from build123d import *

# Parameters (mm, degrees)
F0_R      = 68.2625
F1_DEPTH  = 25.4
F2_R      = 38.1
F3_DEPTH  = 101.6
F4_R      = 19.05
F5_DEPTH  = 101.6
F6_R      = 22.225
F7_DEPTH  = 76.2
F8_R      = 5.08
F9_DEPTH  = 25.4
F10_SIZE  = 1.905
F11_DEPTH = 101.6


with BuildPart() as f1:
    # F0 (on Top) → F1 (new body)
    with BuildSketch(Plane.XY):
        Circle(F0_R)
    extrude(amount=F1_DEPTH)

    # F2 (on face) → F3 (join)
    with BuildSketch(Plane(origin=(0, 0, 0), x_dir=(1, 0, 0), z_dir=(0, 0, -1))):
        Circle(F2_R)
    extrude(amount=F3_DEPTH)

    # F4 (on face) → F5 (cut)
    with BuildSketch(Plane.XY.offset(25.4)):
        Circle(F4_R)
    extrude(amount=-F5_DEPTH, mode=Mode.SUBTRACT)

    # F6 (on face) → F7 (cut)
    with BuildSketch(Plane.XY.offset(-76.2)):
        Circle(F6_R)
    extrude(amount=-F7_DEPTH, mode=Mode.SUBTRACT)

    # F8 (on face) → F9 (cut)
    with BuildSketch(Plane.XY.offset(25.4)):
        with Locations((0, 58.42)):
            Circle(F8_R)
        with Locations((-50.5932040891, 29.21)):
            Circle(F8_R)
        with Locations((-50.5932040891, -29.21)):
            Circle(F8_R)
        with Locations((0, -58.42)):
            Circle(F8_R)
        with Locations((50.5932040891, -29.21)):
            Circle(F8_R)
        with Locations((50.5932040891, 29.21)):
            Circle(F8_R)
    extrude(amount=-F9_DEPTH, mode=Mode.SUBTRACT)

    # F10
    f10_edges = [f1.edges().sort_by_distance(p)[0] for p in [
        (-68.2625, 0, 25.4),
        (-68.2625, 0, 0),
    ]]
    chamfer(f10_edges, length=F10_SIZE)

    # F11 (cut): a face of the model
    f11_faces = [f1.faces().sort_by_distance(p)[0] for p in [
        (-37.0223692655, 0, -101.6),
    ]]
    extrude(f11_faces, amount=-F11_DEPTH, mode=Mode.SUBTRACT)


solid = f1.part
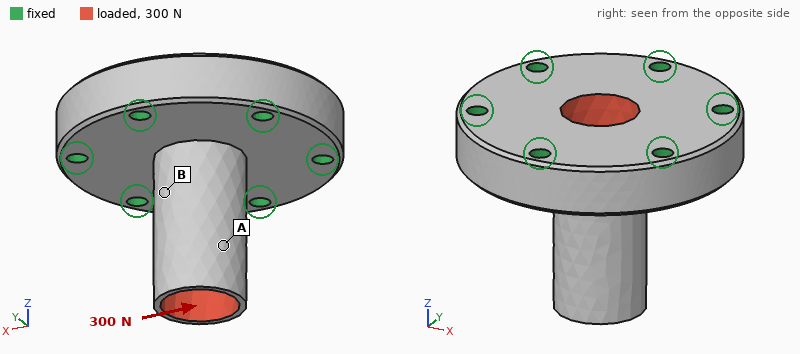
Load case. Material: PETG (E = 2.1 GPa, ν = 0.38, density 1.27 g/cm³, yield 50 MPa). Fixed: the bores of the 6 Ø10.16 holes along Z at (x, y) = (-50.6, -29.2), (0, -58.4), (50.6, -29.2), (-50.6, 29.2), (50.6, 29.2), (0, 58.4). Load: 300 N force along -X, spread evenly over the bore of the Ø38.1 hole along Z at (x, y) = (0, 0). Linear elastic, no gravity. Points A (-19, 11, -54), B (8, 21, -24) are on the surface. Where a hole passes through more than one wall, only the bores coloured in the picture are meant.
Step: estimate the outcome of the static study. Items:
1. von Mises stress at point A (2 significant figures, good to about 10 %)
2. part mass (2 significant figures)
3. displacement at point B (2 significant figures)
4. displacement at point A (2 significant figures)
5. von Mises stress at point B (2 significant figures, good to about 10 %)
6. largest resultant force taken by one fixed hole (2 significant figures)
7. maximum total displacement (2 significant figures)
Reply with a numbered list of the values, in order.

1. 0.36 MPa
2. 460 g
3. 0.055 mm
4. 0.13 mm
5. 1.2 MPa
6. 100 N
7. 0.17 mm
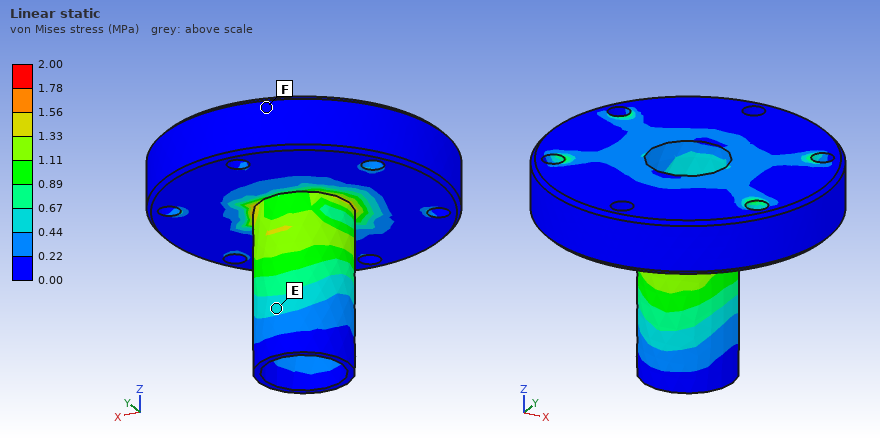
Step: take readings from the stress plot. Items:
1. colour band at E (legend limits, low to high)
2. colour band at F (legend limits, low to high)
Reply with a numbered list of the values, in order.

1. 0.44 to 0.67 MPa
2. 0.00 to 0.22 MPa
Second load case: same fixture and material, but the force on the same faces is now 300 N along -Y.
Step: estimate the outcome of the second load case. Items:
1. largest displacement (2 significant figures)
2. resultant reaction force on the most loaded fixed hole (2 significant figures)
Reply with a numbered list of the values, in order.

1. 0.17 mm
2. 120 N
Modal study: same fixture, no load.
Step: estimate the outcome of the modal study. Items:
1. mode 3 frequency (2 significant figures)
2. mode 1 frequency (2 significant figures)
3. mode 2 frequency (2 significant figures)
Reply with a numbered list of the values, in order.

1. 1400 Hz
2. 1100 Hz
3. 1100 Hz
